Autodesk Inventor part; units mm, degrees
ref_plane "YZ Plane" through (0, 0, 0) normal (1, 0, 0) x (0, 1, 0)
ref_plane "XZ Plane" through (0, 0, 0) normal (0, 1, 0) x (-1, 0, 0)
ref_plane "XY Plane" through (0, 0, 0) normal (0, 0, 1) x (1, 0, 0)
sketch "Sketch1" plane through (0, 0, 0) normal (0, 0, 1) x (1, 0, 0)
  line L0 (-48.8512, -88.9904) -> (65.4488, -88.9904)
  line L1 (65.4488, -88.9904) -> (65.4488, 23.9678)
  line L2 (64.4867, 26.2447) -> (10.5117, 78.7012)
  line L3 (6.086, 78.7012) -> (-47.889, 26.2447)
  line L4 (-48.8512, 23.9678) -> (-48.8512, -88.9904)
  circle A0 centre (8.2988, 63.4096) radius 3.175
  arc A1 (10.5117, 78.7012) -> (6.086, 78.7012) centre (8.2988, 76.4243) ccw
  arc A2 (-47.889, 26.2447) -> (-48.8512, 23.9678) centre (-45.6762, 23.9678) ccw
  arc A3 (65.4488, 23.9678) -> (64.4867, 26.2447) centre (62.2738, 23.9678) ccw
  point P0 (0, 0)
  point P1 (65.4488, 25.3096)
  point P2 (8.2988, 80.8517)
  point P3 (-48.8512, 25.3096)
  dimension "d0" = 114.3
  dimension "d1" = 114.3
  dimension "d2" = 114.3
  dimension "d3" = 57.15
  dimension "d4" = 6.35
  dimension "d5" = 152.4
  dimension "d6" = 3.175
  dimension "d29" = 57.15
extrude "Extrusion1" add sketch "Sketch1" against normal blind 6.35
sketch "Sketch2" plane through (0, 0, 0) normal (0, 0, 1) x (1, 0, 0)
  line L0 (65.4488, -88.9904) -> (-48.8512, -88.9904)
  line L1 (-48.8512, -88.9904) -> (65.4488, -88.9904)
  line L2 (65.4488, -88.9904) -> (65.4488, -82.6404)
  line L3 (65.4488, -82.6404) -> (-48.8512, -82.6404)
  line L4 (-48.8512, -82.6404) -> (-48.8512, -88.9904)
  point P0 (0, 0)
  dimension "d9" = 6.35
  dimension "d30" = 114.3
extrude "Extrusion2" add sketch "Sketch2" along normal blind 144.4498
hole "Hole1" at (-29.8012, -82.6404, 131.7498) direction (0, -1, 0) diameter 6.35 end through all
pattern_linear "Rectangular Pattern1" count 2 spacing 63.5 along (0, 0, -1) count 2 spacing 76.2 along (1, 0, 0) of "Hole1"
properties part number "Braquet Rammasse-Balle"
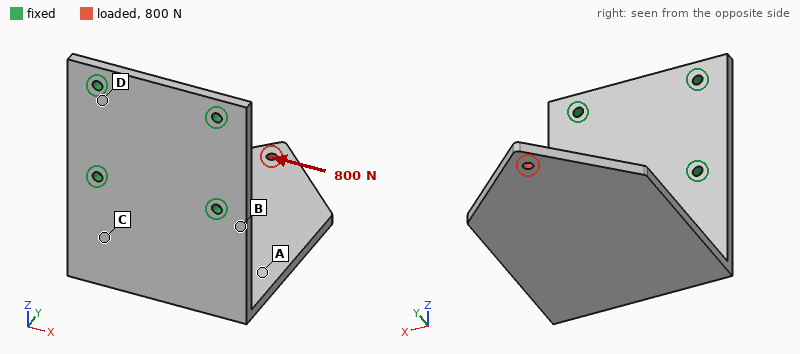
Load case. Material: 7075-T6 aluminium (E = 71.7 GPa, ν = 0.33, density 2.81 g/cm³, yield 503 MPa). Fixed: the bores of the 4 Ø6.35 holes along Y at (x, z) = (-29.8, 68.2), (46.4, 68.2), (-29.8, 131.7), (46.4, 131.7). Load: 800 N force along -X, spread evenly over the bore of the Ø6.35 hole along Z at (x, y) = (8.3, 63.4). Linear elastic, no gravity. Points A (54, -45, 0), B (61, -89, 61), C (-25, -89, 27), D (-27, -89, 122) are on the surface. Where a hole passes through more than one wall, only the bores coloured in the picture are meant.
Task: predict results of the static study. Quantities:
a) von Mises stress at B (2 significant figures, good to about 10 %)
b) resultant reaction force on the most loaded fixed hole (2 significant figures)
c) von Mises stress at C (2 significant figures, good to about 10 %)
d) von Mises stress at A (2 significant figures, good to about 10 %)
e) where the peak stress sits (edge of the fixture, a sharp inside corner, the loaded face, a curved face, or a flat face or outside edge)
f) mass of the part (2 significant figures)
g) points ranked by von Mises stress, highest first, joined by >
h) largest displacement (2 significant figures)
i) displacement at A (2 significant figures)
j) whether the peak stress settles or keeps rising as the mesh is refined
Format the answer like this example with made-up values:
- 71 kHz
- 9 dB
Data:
- 110 MPa
- 1.7 kN
- 80 MPa
- 28 MPa
- edge of the fixture
- 580 g
- B > C > A > D
- 2.7 mm
- 1.0 mm
- keeps rising
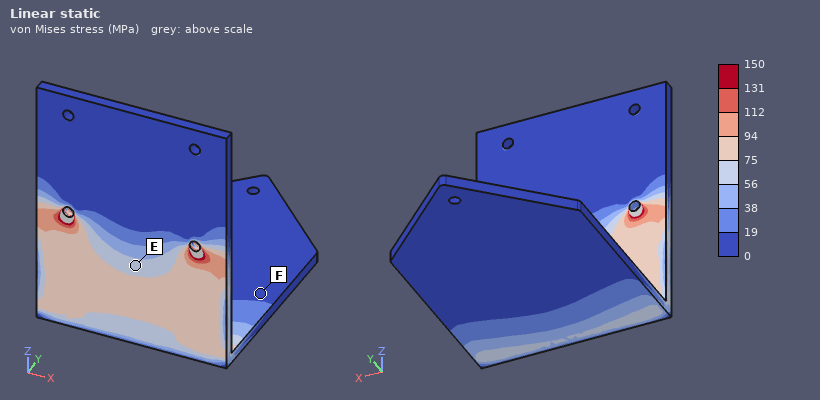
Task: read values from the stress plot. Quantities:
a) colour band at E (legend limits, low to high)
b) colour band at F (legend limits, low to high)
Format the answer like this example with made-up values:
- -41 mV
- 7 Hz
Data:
- 56 to 75 MPa
- 0 to 19 MPa
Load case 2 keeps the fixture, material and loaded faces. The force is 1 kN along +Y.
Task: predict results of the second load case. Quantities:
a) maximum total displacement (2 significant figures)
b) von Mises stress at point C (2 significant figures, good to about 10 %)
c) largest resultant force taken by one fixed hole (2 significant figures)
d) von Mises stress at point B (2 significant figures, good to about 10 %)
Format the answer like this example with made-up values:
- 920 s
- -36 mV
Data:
- 2.6 mm
- 36 MPa
- 680 N
- 74 MPa
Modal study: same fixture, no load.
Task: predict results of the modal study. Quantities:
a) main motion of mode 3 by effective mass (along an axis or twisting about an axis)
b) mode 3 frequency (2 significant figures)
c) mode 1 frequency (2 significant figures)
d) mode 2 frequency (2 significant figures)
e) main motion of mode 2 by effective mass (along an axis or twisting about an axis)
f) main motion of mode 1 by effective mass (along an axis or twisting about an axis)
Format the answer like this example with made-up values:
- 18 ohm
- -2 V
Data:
- along Y
- 480 Hz
- 140 Hz
- 290 Hz
- along X
- along Z
